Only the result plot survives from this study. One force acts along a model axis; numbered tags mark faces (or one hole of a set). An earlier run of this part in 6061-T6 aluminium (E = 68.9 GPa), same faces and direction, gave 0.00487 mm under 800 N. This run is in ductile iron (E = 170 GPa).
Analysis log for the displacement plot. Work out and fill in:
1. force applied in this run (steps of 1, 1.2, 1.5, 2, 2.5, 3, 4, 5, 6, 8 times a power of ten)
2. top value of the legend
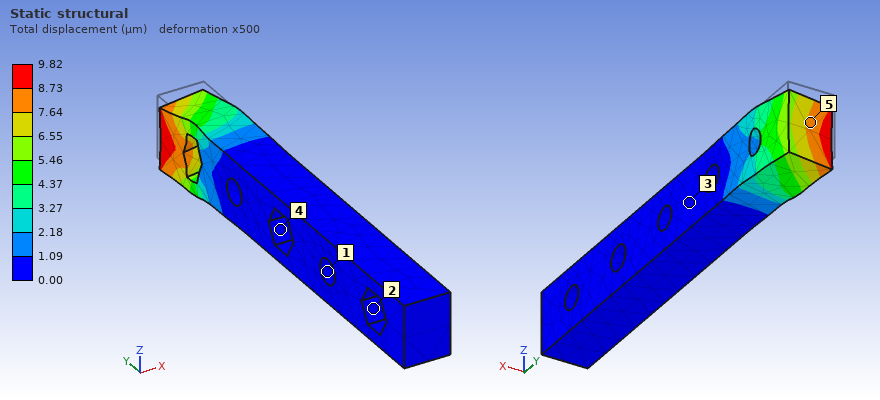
4 kN
9.82 µm
